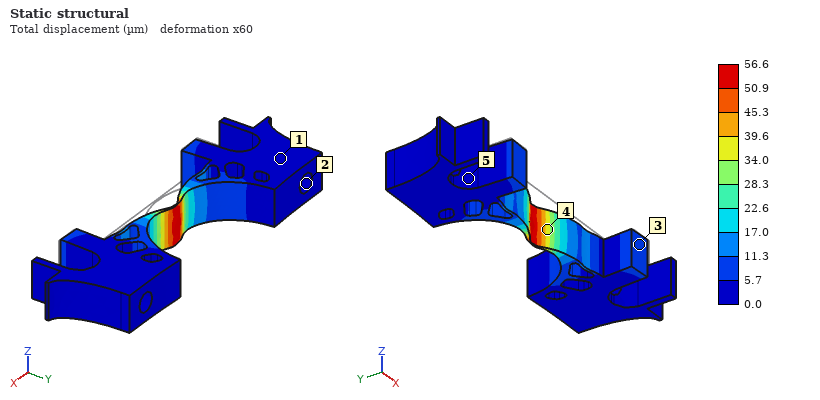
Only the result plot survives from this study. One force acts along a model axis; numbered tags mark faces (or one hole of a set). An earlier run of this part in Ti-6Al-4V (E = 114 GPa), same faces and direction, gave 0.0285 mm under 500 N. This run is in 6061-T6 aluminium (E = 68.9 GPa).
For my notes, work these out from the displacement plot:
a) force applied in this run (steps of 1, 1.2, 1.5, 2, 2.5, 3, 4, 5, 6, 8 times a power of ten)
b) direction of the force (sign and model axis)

600 N
+Y
